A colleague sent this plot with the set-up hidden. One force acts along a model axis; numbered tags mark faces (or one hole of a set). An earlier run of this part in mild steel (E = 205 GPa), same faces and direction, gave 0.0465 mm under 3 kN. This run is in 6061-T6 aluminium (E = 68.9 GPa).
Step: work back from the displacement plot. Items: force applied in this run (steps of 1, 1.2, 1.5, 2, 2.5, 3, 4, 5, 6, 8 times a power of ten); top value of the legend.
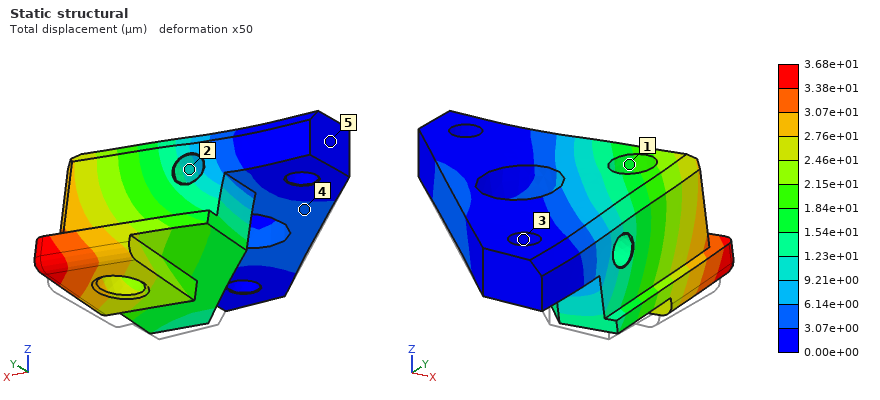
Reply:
800 N
3.68e+01 µm
